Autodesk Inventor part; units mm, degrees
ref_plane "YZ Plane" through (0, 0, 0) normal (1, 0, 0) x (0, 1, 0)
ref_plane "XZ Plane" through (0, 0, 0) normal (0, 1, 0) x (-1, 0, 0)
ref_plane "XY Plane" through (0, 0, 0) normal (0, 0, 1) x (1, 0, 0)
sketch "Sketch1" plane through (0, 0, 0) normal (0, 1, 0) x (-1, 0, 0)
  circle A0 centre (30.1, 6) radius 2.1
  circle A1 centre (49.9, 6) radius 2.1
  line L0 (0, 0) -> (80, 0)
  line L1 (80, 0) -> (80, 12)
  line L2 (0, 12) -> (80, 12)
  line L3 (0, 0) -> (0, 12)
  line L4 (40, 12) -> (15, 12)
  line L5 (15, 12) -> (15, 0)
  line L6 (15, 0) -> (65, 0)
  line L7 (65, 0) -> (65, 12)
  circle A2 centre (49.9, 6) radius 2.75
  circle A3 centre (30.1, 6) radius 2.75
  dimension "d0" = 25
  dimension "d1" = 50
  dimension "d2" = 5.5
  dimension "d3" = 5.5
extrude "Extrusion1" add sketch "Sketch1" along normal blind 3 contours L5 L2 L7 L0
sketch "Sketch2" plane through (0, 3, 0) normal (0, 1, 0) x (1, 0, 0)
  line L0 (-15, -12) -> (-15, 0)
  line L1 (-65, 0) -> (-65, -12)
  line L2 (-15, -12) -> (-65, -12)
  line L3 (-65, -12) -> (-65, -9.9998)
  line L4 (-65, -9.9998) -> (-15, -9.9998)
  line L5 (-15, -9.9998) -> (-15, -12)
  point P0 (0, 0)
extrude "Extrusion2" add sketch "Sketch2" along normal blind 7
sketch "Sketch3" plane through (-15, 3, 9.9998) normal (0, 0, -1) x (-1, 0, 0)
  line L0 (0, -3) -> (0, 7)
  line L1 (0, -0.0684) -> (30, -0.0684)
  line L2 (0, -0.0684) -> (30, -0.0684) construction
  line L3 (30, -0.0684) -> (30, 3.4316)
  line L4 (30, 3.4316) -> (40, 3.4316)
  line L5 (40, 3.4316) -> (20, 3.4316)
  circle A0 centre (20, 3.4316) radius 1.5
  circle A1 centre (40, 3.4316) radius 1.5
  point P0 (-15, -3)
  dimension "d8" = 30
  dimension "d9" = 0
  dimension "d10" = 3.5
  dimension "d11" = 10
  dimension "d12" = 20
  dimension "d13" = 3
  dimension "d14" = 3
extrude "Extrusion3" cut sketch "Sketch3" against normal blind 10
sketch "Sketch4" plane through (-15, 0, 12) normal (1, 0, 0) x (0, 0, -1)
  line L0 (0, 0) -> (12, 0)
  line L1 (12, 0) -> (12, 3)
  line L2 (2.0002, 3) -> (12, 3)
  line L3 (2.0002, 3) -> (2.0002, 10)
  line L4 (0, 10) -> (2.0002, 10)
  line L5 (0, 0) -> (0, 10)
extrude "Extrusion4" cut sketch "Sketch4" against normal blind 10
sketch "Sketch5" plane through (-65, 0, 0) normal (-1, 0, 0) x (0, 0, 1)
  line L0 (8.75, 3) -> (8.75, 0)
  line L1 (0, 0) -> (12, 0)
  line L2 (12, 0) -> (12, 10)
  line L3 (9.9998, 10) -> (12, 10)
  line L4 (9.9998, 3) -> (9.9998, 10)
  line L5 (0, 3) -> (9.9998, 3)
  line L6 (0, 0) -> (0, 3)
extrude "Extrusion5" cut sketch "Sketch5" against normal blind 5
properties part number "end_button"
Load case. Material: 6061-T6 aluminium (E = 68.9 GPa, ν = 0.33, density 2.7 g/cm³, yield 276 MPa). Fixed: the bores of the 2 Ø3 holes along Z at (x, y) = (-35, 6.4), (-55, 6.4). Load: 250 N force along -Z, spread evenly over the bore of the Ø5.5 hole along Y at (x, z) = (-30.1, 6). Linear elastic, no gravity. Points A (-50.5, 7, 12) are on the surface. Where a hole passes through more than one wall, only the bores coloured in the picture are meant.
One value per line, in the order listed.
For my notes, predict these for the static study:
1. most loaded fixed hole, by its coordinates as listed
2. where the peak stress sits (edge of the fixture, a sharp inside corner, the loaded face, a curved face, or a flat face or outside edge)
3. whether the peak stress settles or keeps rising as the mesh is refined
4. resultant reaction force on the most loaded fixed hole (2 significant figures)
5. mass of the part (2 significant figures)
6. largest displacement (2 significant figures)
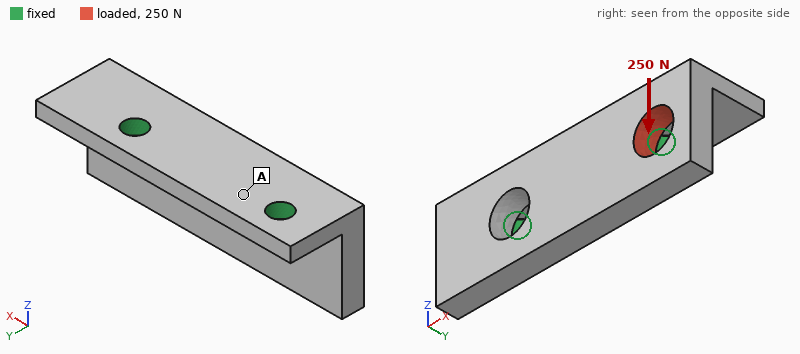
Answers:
(-35, 6.4)
edge of the fixture
keeps rising
300 N
4.3 g
49 µm
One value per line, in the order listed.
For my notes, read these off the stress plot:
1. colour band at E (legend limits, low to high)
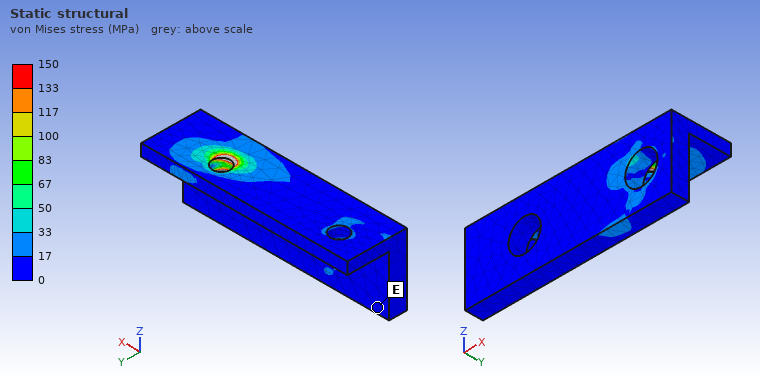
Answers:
0 to 17 MPa
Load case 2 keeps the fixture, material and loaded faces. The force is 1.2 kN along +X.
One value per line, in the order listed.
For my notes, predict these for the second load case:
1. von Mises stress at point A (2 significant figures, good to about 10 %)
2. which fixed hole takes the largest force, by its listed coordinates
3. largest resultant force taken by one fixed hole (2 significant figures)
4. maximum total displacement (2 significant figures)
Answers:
23 MPa
(-35, 6.4)
780 N
40 µm
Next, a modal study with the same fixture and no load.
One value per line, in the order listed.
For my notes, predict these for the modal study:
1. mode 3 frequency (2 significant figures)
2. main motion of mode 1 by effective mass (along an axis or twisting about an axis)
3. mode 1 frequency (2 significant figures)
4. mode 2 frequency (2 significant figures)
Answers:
20 kHz
along Y
7400 Hz
12 kHz
